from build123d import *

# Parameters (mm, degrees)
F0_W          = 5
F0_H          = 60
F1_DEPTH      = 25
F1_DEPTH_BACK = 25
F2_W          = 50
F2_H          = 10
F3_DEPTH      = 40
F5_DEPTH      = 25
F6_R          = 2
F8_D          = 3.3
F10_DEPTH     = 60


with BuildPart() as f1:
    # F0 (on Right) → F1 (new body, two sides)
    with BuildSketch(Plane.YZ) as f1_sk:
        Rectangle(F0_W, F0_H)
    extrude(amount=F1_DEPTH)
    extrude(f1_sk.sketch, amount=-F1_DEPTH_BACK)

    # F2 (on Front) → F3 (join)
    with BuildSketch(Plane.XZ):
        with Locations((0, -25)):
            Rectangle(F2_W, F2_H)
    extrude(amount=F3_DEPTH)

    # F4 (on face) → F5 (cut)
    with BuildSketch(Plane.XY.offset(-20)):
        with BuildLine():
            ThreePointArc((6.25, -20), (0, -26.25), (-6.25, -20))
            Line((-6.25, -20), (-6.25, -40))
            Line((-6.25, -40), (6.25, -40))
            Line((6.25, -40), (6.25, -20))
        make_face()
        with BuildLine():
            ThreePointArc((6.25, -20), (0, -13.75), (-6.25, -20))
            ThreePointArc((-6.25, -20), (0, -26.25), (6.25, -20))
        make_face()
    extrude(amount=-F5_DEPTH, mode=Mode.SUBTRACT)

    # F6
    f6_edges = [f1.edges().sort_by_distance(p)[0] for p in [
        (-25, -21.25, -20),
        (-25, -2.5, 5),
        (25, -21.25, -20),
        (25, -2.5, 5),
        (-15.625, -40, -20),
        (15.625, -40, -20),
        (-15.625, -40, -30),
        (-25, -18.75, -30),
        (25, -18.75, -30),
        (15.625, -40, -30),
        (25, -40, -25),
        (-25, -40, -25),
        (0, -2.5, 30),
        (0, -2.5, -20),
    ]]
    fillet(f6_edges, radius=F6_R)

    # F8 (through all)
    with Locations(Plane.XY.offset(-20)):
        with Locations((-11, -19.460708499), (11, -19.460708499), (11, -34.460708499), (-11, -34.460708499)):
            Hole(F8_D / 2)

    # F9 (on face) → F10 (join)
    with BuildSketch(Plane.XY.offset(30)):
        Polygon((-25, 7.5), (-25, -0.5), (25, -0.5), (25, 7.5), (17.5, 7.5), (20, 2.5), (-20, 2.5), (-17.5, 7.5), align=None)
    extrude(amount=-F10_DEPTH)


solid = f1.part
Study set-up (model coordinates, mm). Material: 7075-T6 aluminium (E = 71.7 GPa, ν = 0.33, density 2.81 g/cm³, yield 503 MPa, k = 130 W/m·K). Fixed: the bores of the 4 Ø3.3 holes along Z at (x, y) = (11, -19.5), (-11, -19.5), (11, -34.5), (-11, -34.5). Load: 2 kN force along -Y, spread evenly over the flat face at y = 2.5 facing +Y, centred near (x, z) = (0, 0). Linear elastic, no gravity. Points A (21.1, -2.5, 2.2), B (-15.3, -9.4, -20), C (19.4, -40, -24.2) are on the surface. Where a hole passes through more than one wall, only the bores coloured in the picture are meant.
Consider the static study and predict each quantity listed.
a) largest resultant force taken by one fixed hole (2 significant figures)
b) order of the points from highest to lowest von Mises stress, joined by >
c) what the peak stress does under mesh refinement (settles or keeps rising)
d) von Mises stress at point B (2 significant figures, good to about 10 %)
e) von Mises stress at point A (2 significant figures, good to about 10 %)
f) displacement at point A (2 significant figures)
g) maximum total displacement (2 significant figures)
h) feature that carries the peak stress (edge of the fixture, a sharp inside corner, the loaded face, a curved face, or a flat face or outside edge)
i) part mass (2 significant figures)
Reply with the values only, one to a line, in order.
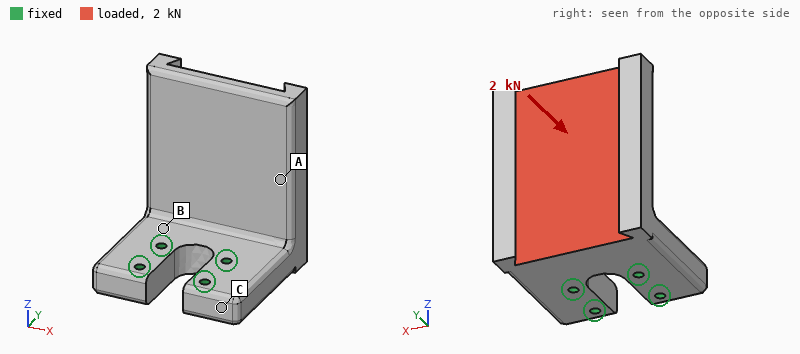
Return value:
1.0 kN
B > A > C
keeps rising
69 MPa
29 MPa
0.21 mm
0.53 mm
edge of the fixture
95 g
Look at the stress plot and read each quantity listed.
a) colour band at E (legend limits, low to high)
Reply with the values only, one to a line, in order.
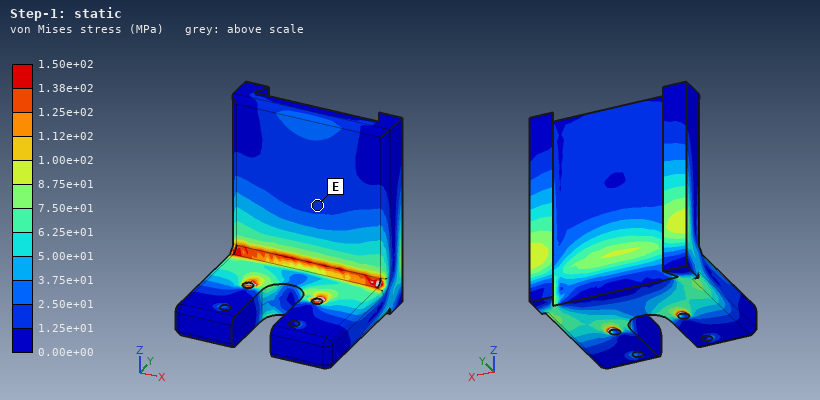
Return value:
1.25e+01 to 2.50e+01 MPa
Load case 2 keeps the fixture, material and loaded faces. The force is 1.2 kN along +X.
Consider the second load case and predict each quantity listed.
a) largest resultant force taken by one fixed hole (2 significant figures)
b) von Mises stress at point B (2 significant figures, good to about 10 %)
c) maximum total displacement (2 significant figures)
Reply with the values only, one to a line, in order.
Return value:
1.4 kN
19 MPa
67 µm
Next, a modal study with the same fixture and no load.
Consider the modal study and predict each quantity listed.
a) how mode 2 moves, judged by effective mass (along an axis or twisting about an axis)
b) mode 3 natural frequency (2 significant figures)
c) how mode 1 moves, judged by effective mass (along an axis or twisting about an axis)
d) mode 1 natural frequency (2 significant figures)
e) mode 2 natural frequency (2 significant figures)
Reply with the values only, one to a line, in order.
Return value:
along X
3800 Hz
along Y
1700 Hz
3000 Hz
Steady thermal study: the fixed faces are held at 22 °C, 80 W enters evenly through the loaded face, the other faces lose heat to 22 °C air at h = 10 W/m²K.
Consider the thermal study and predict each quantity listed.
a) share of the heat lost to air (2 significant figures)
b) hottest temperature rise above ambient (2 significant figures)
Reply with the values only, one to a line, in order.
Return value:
4.3 %
73 K
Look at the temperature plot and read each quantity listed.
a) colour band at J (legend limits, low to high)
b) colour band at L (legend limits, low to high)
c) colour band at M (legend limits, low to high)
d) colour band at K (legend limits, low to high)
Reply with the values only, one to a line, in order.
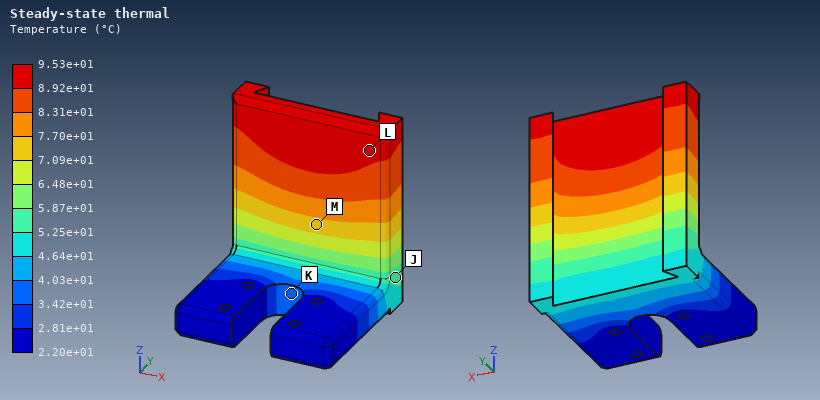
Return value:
5.25e+01 to 5.87e+01 °C
8.92e+01 to 9.53e+01 °C
7.09e+01 to 7.70e+01 °C
3.42e+01 to 4.03e+01 °C
